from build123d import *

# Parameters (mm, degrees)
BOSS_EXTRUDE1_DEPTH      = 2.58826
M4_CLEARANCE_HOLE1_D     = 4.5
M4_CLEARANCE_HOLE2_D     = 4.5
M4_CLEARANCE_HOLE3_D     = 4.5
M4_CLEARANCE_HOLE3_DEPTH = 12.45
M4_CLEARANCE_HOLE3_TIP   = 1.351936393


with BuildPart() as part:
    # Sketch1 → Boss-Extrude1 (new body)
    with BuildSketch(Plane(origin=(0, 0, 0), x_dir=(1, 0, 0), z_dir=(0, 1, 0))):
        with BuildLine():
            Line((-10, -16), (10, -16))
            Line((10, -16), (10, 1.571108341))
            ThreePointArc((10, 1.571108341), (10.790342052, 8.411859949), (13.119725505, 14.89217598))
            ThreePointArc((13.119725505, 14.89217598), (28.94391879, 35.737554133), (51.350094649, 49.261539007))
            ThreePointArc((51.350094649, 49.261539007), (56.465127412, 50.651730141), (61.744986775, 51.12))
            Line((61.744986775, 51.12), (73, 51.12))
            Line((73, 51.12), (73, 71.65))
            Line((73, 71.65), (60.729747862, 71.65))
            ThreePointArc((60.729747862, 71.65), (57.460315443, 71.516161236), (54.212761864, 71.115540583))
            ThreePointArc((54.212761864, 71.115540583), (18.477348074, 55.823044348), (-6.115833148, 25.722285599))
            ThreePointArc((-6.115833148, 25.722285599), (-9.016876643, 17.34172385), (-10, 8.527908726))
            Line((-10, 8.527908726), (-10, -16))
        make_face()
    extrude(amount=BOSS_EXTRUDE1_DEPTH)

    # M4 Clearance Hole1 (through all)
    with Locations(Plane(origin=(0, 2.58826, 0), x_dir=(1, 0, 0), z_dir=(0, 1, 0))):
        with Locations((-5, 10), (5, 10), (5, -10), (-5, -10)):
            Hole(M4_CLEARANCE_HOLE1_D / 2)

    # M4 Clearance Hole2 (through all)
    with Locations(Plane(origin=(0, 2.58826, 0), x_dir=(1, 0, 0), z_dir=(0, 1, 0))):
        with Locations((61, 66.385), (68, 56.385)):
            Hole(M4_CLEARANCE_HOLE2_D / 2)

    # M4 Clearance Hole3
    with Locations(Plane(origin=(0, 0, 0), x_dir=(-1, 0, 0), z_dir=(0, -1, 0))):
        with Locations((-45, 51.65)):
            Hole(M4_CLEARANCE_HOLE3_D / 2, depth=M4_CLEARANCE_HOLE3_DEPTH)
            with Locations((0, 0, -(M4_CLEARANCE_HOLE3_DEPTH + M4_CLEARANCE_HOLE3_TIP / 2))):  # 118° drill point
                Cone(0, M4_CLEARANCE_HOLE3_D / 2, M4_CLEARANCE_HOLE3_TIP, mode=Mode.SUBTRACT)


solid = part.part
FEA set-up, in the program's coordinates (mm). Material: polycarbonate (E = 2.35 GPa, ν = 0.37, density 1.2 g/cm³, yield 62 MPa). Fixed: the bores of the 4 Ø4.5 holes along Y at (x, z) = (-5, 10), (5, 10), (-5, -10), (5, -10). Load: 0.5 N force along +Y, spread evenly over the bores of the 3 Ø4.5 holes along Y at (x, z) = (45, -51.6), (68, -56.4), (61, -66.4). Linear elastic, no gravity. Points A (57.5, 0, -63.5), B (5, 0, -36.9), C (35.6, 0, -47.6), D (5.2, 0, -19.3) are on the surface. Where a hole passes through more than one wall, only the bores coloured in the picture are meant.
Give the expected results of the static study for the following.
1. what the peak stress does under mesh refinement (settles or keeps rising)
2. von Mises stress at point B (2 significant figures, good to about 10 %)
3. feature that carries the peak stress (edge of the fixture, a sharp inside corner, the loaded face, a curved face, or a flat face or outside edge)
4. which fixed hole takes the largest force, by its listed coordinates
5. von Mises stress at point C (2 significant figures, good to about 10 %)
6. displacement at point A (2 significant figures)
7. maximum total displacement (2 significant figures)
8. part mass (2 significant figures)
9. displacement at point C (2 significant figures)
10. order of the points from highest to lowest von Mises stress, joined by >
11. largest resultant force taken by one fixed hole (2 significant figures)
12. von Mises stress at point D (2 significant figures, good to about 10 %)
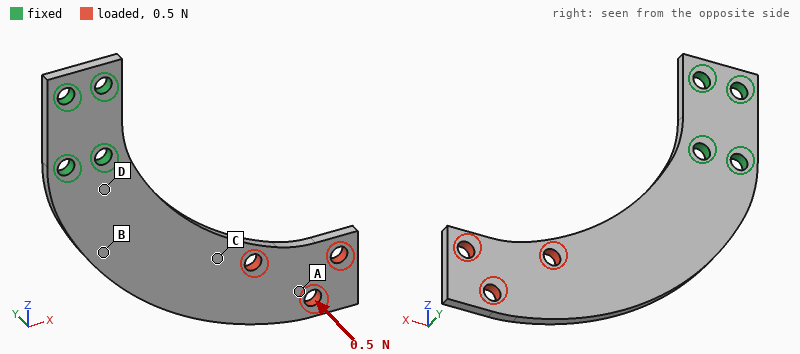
keeps rising
0.96 MPa
edge of the fixture
(5, -10)
0.56 MPa
0.91 mm
1.2 mm
7.7 g
0.44 mm
D > B > C > A
2.3 N
1.2 MPa
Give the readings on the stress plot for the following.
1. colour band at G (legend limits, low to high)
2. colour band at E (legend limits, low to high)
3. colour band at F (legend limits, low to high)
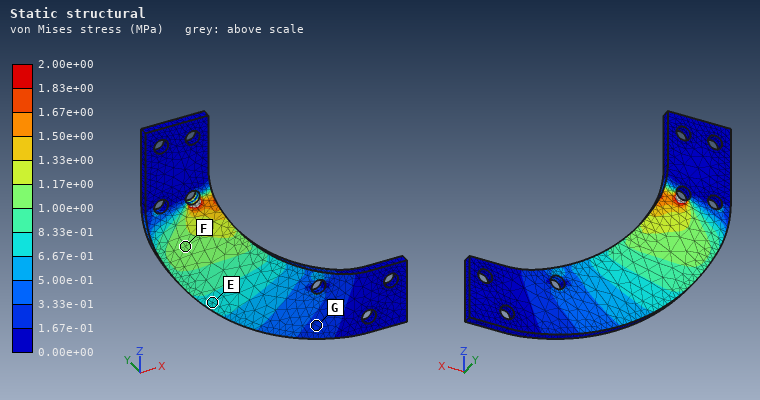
1.67e-01 to 3.33e-01 MPa
6.67e-01 to 8.33e-01 MPa
1.00e+00 to 1.17e+00 MPa
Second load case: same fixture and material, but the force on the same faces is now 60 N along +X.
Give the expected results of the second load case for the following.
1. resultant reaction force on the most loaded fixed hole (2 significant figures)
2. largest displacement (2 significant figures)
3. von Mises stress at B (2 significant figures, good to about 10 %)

210 N
1.4 mm
5.5 MPa
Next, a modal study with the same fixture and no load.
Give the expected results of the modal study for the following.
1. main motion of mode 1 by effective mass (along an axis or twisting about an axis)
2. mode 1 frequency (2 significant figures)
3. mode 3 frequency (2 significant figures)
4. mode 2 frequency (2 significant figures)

along Y
76 Hz
550 Hz
330 Hz
